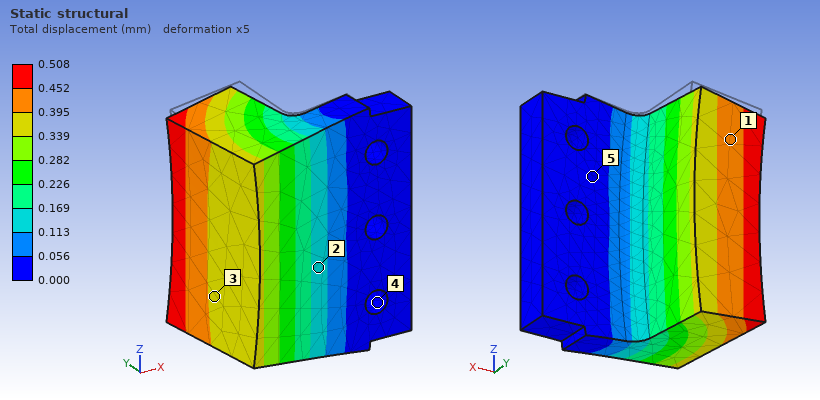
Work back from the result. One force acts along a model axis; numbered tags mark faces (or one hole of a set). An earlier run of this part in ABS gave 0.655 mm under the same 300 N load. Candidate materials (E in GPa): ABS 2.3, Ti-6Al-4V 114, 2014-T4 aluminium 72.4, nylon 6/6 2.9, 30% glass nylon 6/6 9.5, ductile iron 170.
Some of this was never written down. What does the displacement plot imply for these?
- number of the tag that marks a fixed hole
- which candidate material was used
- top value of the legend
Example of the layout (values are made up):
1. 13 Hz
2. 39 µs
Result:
1. 4
2. nylon 6/6
3. 0.508 mm
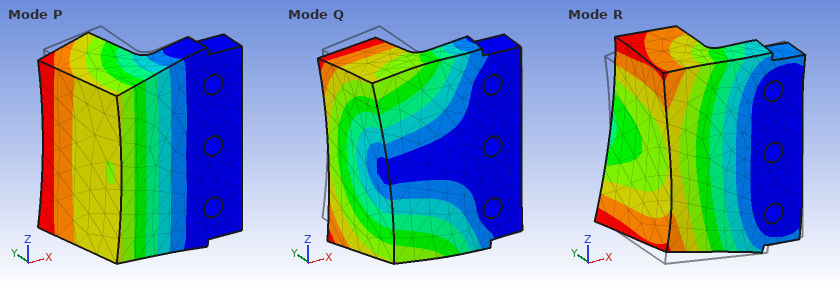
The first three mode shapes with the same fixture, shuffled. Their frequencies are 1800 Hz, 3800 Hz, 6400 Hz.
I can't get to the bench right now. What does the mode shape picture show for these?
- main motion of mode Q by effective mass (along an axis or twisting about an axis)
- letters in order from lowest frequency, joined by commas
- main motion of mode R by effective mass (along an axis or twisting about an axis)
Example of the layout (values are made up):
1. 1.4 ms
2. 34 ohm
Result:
1. along Z
2. P, Q, R
3. along Z
